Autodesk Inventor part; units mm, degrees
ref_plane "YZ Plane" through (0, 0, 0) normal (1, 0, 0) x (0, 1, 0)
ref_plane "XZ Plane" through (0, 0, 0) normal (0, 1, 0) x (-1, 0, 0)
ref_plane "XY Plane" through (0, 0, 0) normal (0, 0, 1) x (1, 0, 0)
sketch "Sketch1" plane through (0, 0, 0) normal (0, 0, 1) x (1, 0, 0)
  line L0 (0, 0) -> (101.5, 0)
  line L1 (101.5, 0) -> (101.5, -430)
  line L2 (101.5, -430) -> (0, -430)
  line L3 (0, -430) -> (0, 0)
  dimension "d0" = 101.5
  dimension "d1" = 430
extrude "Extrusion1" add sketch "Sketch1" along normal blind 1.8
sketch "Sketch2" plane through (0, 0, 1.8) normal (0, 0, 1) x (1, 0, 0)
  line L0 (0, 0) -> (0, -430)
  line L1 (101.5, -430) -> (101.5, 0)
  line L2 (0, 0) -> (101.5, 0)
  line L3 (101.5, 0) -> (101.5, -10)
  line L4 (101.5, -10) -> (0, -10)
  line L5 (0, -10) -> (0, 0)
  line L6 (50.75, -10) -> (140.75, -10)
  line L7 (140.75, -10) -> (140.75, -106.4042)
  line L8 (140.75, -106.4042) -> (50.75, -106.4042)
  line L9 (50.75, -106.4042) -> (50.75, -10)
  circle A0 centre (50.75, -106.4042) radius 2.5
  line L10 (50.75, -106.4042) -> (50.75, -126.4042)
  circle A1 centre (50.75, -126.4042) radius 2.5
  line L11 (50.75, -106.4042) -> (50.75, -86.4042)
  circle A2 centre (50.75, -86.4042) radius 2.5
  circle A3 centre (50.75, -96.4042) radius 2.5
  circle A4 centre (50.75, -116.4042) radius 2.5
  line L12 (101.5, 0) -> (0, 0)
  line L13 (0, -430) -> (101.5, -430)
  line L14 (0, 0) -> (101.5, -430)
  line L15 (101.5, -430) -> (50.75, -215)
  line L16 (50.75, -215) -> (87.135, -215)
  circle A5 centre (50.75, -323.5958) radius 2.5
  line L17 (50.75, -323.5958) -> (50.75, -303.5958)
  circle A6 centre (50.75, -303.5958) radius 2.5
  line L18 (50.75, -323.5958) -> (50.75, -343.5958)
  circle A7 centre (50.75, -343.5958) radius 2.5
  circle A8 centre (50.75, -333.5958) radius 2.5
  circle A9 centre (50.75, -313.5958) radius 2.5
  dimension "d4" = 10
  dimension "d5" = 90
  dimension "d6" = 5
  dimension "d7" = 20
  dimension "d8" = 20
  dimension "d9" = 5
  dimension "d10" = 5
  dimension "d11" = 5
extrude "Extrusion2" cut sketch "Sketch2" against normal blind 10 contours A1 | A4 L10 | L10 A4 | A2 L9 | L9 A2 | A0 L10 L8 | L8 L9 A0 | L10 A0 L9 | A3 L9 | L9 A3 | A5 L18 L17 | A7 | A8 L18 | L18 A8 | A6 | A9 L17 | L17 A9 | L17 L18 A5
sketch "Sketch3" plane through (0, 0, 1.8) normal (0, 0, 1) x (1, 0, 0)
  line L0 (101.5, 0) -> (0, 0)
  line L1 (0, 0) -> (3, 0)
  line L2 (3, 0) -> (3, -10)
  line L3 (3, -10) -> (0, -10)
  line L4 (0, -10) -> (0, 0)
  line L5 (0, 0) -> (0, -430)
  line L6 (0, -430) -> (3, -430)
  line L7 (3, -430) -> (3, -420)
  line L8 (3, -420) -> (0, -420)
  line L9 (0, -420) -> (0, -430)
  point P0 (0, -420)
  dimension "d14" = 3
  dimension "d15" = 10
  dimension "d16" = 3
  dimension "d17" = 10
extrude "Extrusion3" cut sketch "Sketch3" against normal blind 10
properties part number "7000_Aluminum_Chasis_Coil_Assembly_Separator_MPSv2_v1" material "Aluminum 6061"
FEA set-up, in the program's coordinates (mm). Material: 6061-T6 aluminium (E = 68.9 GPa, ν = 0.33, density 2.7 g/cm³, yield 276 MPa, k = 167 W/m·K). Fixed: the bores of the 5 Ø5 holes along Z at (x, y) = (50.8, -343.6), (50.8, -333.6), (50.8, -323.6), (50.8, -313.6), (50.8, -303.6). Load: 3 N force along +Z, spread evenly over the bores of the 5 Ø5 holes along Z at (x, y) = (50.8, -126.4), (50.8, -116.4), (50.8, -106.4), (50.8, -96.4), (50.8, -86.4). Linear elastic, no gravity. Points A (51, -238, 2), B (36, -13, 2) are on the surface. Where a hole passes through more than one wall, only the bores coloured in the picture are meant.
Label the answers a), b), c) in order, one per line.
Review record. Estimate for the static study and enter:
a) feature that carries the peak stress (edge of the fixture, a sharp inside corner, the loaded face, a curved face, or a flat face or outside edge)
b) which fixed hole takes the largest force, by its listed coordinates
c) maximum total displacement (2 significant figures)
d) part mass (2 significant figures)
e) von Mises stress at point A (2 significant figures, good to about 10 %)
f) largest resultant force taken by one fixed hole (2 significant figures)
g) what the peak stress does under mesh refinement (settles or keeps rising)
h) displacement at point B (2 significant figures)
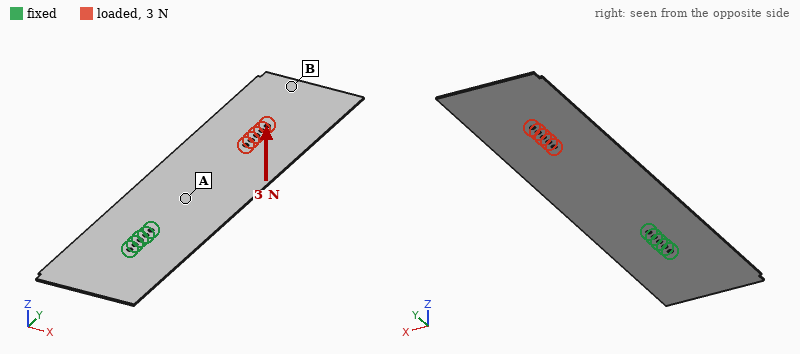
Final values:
a) edge of the fixture
b) (50.8, -303.6)
c) 4.2 mm
d) 210 g
e) 6.6 MPa
f) 23 N
g) keeps rising
h) 4.0 mm
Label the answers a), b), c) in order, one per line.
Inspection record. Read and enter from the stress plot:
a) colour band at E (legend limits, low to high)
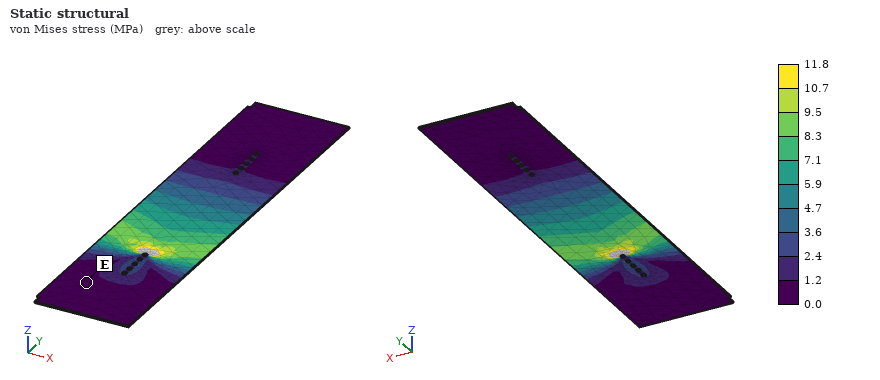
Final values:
a) 0.0 to 1.2 MPa
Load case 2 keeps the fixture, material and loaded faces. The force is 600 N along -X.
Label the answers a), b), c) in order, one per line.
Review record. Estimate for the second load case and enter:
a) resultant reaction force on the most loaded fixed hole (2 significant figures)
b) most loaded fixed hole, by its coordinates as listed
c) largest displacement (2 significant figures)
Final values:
a) 2.9 kN
b) (50.8, -303.6)
c) 0.70 mm
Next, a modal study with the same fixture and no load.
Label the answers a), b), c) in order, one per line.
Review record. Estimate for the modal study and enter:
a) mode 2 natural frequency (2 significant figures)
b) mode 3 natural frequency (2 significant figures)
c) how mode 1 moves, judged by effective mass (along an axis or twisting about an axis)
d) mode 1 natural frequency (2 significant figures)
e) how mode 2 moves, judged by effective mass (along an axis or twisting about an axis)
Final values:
a) 89 Hz
b) 97 Hz
c) along Z
d) 16 Hz
e) twisting about Y
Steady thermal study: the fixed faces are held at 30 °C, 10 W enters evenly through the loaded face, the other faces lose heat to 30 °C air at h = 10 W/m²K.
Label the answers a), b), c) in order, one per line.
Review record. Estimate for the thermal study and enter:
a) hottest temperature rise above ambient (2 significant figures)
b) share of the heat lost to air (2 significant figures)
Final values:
a) 26 K
b) 81 %
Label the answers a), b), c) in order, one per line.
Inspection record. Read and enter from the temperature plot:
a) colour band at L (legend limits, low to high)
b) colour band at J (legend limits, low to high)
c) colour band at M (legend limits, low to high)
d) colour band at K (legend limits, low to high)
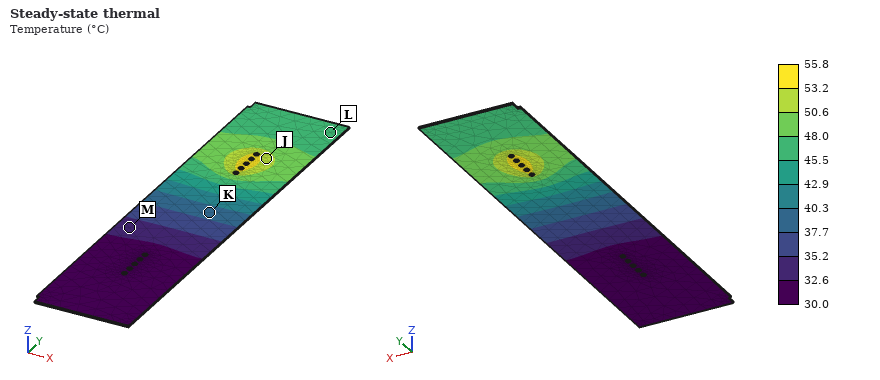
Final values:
a) 45.5 to 48.0 °C
b) 50.6 to 53.2 °C
c) 32.6 to 35.2 °C
d) 37.7 to 40.3 °C
